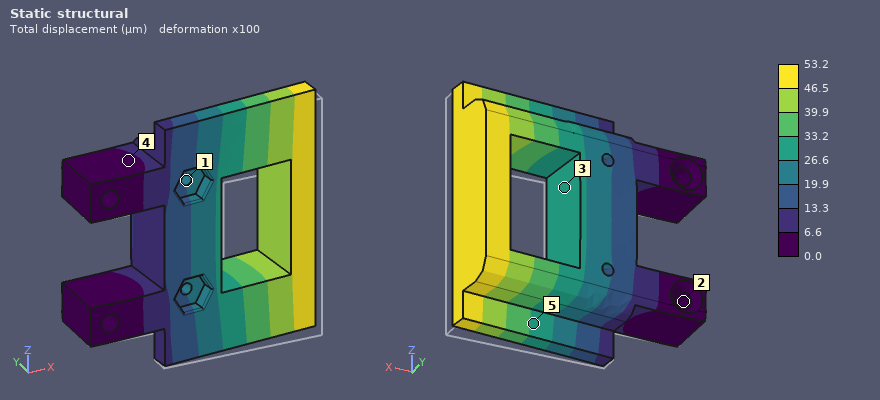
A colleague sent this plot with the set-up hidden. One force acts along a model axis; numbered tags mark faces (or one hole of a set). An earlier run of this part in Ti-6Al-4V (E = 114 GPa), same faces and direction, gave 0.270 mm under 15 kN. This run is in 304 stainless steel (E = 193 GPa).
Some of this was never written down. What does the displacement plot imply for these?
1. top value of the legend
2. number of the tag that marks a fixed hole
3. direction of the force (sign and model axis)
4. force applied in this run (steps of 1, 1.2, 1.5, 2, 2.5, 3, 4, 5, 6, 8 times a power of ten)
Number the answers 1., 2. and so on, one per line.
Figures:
1. 53.2 µm
2. 2
3. +Y
4. 5 kN
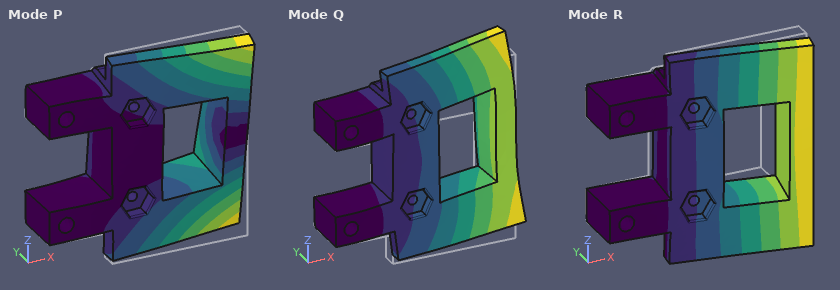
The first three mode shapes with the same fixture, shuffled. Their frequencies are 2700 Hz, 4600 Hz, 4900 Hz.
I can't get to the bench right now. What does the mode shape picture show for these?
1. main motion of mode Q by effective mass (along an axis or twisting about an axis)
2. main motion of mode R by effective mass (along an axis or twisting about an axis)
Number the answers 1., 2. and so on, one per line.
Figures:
1. along Z
2. along Y
